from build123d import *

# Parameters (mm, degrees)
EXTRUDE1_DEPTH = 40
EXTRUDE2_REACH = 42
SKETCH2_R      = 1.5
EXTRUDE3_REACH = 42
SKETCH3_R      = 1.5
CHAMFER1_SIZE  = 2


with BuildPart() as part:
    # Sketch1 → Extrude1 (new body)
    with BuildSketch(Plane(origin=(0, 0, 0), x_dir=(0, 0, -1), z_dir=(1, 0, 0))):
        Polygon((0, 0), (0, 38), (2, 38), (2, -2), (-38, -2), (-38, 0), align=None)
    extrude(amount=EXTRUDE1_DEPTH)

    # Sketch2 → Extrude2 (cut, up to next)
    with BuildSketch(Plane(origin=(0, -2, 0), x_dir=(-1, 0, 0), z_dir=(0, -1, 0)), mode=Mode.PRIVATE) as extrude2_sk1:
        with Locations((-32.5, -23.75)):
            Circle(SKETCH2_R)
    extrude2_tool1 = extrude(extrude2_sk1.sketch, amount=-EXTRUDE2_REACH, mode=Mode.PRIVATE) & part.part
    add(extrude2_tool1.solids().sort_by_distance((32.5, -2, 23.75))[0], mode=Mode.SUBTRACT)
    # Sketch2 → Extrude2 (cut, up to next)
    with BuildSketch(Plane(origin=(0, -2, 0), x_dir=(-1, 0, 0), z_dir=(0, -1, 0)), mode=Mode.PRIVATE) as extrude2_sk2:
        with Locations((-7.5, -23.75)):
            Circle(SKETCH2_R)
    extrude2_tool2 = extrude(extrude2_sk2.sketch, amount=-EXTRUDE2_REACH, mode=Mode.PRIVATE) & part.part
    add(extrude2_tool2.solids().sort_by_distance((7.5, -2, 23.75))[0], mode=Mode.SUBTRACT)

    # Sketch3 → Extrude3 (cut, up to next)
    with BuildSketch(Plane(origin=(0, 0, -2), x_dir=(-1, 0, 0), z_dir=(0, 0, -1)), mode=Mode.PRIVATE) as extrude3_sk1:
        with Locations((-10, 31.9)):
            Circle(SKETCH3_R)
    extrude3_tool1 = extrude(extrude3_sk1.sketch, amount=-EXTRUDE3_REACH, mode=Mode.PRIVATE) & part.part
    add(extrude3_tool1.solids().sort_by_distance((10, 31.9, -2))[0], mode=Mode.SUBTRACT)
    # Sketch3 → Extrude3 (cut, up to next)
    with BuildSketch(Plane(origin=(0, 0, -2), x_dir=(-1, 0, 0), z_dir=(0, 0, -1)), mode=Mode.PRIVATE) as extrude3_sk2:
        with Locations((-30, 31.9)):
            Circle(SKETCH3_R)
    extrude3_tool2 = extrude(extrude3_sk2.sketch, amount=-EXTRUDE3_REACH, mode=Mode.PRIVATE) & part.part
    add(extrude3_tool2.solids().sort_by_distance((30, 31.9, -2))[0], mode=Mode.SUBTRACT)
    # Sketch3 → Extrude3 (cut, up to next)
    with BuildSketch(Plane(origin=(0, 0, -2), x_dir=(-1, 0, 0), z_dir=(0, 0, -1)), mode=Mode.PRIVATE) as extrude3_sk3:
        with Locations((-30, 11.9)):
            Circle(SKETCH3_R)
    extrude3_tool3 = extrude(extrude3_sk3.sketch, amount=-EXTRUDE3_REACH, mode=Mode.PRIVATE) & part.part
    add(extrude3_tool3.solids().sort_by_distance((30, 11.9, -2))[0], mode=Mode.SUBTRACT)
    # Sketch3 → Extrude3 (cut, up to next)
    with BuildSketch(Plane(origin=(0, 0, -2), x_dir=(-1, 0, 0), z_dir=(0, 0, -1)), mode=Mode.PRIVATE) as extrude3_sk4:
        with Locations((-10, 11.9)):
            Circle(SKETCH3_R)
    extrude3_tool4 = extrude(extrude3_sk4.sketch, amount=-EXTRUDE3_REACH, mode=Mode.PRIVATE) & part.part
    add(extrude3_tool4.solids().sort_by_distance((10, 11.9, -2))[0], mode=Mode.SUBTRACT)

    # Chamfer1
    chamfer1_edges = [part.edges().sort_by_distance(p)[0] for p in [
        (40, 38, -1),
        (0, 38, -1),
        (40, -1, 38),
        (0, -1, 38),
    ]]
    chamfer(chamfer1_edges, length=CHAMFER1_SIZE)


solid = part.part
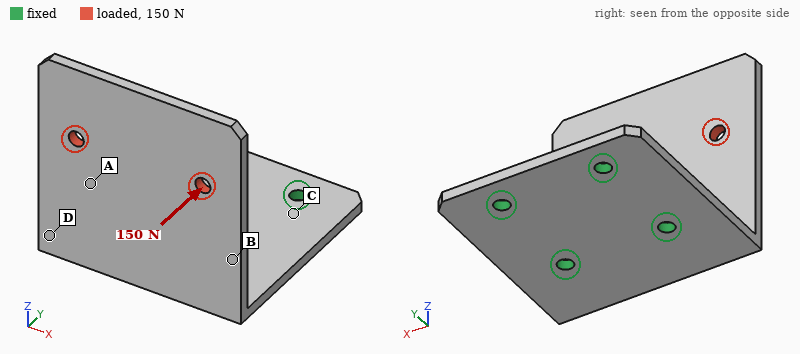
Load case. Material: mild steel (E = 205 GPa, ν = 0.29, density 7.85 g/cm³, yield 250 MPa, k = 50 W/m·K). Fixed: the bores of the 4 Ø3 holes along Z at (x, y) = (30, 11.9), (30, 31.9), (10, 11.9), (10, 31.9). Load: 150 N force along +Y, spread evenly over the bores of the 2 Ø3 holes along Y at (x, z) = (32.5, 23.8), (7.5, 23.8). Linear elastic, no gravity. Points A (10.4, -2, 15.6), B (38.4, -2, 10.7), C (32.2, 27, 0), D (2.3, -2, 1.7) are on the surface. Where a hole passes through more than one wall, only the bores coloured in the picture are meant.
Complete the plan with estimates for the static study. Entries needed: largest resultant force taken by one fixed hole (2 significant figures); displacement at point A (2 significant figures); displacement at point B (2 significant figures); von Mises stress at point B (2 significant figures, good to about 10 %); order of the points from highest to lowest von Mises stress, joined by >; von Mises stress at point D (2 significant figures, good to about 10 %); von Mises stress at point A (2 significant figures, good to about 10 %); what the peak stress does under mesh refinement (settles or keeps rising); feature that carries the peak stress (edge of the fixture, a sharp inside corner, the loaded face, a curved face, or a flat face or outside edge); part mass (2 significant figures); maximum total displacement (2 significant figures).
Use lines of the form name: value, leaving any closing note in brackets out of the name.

largest resultant force taken by one fixed hole: 69 N
displacement at point A: 0.21 mm
displacement at point B: 0.15 mm
von Mises stress at point B: 75 MPa
order of the points from highest to lowest von Mises stress, joined by >: D > B > A > C
von Mises stress at point D: 110 MPa
von Mises stress at point A: 43 MPa
what the peak stress does under mesh refinement: keeps rising
feature that carries the peak stress: edge of the fixture
part mass: 48 g
maximum total displacement: 0.56 mm
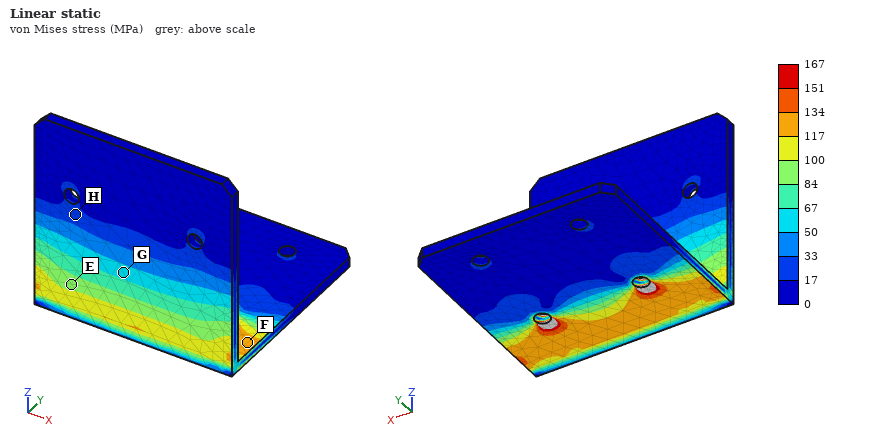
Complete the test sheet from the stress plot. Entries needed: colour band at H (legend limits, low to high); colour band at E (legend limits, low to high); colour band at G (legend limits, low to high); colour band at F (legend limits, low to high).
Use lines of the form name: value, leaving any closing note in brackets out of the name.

colour band at H: 17 to 33 MPa
colour band at E: 84 to 100 MPa
colour band at G: 50 to 67 MPa
colour band at F: 117 to 134 MPa
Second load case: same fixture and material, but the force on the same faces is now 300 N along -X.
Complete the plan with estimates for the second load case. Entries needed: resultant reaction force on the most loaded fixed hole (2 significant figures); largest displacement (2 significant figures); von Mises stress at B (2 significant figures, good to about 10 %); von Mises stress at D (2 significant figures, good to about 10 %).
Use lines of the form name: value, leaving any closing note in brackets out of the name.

resultant reaction force on the most loaded fixed hole: 380 N
largest displacement: 0.16 mm
von Mises stress at B: 31 MPa
von Mises stress at D: 69 MPa
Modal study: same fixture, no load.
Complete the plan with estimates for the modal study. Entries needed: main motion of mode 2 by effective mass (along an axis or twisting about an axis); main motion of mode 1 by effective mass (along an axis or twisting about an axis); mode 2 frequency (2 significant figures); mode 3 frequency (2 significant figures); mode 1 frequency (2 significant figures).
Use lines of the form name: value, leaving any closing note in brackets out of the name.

main motion of mode 2 by effective mass: along X
main motion of mode 1 by effective mass: along Y
mode 2 frequency: 1700 Hz
mode 3 frequency: 2600 Hz
mode 1 frequency: 730 Hz
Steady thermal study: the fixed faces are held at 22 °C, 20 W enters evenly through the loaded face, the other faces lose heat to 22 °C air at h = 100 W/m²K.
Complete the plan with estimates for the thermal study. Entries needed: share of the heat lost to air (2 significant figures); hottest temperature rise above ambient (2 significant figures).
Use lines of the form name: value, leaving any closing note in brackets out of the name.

share of the heat lost to air: 80 %
hottest temperature rise above ambient: 82 K
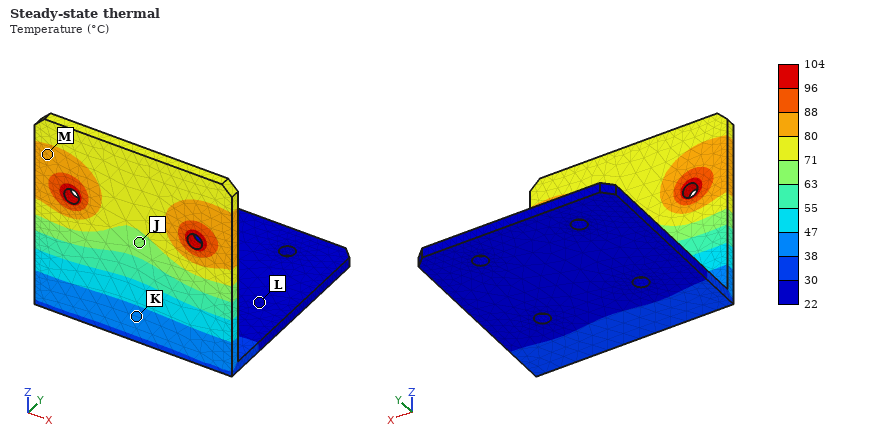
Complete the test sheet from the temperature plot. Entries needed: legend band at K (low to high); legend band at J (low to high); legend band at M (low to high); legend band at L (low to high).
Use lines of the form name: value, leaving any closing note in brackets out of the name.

legend band at K: 38 to 47 °C
legend band at J: 63 to 71 °C
legend band at M: 80 to 88 °C
legend band at L: 22 to 30 °C
